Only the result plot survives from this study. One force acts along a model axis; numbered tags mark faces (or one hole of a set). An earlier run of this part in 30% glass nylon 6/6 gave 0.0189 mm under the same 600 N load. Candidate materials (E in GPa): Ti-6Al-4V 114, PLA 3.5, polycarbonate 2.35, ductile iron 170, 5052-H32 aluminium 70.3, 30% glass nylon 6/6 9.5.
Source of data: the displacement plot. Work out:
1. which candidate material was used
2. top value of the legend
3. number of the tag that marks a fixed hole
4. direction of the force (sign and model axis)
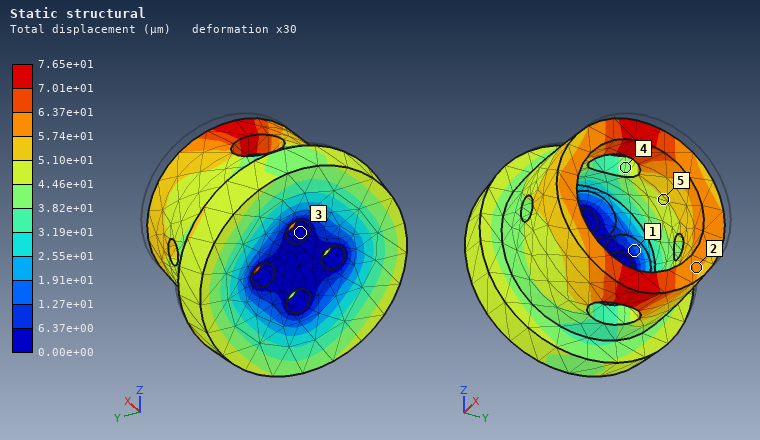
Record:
polycarbonate
7.65e+01 µm
3
-X
